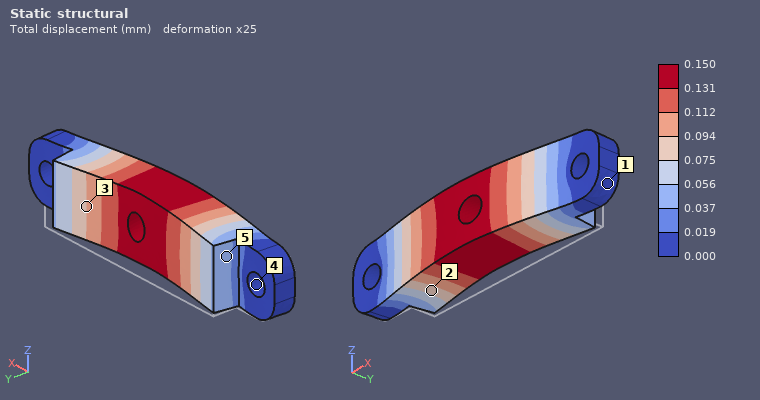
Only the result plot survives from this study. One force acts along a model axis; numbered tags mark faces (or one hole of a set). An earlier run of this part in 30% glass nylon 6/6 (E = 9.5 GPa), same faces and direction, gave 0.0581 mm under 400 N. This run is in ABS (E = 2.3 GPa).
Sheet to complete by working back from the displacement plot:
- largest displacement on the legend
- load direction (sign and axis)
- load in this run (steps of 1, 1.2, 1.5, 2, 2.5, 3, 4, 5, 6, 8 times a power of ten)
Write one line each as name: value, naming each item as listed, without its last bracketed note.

largest displacement on the legend: 0.150 mm
load direction: -Y
load in this run: 250 N
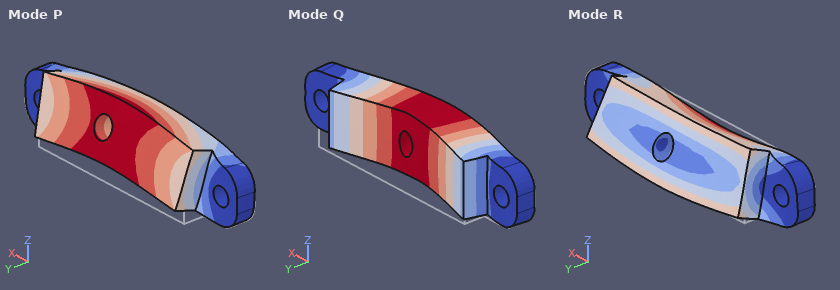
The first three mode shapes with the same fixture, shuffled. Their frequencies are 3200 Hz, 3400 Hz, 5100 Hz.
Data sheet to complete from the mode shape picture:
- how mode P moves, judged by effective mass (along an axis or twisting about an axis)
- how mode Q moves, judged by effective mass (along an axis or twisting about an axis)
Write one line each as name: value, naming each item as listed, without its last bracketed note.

how mode P moves, judged by effective mass: along Z
how mode Q moves, judged by effective mass: along Y
